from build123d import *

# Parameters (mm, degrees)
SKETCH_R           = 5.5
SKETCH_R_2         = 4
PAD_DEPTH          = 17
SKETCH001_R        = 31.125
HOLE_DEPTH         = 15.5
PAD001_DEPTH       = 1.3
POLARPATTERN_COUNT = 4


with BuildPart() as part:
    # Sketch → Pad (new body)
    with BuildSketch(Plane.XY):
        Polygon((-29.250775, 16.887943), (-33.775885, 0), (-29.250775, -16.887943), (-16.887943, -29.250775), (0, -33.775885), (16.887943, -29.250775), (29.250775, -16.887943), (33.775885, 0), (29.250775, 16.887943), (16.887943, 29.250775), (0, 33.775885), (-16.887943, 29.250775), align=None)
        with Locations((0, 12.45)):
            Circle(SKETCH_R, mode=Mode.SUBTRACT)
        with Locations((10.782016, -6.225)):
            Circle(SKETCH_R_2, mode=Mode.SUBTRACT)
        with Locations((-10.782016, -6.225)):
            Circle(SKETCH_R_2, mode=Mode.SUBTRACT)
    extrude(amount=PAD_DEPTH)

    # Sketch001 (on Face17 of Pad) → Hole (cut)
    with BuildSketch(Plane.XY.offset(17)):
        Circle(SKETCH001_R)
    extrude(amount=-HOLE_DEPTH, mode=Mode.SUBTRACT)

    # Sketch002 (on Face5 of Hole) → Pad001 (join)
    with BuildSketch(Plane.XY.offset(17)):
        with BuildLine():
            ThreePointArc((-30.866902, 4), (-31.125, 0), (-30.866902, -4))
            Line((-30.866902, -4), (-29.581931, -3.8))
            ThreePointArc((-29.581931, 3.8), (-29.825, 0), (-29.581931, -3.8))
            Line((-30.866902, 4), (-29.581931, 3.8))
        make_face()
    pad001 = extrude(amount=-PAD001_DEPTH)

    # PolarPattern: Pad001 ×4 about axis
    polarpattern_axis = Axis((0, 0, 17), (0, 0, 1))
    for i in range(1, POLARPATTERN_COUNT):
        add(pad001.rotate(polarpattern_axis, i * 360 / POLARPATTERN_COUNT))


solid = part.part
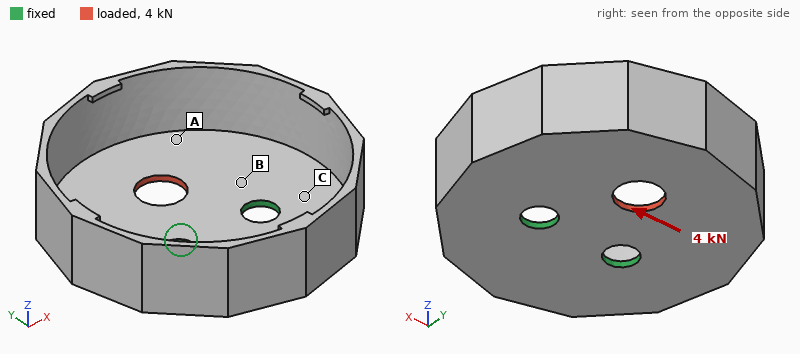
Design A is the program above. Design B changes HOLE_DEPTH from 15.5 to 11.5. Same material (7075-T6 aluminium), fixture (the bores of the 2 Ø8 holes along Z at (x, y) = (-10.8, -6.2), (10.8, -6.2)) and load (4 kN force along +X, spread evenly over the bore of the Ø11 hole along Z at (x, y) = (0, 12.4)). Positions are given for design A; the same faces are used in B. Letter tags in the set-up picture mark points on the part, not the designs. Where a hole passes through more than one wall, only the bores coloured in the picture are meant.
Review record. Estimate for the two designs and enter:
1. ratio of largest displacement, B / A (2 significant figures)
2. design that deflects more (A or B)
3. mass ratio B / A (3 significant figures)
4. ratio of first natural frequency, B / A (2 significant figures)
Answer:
0.25
A
2.06
4.0
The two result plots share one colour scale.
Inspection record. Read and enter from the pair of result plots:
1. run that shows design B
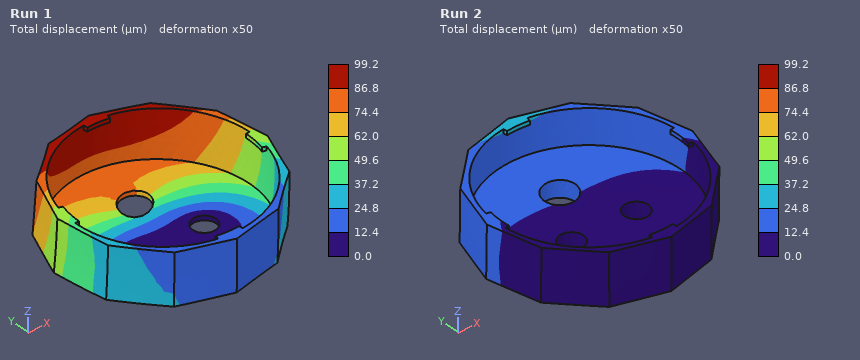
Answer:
Run 2
